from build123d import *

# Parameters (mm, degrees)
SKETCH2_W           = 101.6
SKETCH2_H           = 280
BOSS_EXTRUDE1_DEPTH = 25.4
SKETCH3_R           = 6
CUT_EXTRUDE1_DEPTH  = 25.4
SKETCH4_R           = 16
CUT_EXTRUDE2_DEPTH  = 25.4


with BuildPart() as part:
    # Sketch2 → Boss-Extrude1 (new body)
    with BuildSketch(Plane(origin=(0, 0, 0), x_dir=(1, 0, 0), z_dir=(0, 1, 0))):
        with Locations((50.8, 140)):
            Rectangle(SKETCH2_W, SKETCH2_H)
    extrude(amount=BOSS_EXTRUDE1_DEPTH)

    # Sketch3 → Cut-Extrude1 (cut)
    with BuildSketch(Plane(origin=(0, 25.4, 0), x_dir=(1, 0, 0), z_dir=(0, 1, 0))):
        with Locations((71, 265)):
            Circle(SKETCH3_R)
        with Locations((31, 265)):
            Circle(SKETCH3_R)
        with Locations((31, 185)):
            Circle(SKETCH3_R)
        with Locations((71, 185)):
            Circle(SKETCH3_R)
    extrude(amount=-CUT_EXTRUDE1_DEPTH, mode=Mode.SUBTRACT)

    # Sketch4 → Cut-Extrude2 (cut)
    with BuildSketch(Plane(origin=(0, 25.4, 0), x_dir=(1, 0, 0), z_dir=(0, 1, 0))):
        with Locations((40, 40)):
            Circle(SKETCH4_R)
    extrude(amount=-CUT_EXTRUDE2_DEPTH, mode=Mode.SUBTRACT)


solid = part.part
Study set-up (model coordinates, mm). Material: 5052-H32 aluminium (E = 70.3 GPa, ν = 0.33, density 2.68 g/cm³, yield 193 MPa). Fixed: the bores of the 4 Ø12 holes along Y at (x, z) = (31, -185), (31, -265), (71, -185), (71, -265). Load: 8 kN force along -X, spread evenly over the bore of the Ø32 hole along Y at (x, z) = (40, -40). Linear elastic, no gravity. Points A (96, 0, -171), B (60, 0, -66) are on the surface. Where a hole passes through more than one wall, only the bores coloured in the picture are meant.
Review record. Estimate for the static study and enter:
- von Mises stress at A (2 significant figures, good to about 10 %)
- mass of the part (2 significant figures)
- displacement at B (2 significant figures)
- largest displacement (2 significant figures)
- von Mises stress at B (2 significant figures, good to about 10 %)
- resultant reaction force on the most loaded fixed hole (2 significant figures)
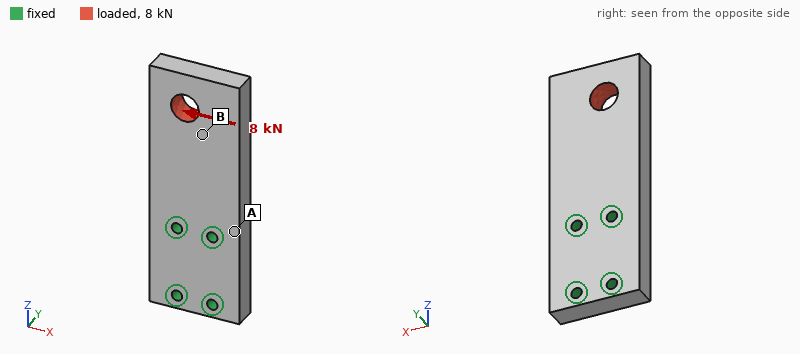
17 MPa
1.9 kg
0.071 mm
0.13 mm
6.6 MPa
17 kN
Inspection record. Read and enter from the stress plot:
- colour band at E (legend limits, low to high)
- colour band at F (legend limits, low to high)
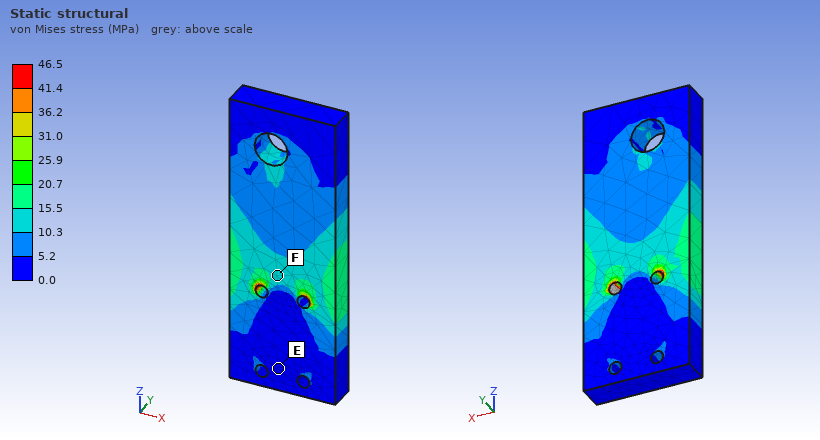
0.0 to 5.2 MPa
10.3 to 15.5 MPa
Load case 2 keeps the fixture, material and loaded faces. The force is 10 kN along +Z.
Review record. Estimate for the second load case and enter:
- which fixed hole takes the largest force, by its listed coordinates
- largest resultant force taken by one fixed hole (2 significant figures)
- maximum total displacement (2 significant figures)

(31, -185)
6.0 kN
19 µm
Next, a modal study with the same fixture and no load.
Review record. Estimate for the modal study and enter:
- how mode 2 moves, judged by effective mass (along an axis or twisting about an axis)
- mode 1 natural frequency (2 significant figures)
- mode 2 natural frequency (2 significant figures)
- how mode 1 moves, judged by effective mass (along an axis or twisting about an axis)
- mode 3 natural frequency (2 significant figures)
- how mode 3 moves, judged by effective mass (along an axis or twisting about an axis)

along X
630 Hz
1800 Hz
along Y
2000 Hz
twisting about Z
